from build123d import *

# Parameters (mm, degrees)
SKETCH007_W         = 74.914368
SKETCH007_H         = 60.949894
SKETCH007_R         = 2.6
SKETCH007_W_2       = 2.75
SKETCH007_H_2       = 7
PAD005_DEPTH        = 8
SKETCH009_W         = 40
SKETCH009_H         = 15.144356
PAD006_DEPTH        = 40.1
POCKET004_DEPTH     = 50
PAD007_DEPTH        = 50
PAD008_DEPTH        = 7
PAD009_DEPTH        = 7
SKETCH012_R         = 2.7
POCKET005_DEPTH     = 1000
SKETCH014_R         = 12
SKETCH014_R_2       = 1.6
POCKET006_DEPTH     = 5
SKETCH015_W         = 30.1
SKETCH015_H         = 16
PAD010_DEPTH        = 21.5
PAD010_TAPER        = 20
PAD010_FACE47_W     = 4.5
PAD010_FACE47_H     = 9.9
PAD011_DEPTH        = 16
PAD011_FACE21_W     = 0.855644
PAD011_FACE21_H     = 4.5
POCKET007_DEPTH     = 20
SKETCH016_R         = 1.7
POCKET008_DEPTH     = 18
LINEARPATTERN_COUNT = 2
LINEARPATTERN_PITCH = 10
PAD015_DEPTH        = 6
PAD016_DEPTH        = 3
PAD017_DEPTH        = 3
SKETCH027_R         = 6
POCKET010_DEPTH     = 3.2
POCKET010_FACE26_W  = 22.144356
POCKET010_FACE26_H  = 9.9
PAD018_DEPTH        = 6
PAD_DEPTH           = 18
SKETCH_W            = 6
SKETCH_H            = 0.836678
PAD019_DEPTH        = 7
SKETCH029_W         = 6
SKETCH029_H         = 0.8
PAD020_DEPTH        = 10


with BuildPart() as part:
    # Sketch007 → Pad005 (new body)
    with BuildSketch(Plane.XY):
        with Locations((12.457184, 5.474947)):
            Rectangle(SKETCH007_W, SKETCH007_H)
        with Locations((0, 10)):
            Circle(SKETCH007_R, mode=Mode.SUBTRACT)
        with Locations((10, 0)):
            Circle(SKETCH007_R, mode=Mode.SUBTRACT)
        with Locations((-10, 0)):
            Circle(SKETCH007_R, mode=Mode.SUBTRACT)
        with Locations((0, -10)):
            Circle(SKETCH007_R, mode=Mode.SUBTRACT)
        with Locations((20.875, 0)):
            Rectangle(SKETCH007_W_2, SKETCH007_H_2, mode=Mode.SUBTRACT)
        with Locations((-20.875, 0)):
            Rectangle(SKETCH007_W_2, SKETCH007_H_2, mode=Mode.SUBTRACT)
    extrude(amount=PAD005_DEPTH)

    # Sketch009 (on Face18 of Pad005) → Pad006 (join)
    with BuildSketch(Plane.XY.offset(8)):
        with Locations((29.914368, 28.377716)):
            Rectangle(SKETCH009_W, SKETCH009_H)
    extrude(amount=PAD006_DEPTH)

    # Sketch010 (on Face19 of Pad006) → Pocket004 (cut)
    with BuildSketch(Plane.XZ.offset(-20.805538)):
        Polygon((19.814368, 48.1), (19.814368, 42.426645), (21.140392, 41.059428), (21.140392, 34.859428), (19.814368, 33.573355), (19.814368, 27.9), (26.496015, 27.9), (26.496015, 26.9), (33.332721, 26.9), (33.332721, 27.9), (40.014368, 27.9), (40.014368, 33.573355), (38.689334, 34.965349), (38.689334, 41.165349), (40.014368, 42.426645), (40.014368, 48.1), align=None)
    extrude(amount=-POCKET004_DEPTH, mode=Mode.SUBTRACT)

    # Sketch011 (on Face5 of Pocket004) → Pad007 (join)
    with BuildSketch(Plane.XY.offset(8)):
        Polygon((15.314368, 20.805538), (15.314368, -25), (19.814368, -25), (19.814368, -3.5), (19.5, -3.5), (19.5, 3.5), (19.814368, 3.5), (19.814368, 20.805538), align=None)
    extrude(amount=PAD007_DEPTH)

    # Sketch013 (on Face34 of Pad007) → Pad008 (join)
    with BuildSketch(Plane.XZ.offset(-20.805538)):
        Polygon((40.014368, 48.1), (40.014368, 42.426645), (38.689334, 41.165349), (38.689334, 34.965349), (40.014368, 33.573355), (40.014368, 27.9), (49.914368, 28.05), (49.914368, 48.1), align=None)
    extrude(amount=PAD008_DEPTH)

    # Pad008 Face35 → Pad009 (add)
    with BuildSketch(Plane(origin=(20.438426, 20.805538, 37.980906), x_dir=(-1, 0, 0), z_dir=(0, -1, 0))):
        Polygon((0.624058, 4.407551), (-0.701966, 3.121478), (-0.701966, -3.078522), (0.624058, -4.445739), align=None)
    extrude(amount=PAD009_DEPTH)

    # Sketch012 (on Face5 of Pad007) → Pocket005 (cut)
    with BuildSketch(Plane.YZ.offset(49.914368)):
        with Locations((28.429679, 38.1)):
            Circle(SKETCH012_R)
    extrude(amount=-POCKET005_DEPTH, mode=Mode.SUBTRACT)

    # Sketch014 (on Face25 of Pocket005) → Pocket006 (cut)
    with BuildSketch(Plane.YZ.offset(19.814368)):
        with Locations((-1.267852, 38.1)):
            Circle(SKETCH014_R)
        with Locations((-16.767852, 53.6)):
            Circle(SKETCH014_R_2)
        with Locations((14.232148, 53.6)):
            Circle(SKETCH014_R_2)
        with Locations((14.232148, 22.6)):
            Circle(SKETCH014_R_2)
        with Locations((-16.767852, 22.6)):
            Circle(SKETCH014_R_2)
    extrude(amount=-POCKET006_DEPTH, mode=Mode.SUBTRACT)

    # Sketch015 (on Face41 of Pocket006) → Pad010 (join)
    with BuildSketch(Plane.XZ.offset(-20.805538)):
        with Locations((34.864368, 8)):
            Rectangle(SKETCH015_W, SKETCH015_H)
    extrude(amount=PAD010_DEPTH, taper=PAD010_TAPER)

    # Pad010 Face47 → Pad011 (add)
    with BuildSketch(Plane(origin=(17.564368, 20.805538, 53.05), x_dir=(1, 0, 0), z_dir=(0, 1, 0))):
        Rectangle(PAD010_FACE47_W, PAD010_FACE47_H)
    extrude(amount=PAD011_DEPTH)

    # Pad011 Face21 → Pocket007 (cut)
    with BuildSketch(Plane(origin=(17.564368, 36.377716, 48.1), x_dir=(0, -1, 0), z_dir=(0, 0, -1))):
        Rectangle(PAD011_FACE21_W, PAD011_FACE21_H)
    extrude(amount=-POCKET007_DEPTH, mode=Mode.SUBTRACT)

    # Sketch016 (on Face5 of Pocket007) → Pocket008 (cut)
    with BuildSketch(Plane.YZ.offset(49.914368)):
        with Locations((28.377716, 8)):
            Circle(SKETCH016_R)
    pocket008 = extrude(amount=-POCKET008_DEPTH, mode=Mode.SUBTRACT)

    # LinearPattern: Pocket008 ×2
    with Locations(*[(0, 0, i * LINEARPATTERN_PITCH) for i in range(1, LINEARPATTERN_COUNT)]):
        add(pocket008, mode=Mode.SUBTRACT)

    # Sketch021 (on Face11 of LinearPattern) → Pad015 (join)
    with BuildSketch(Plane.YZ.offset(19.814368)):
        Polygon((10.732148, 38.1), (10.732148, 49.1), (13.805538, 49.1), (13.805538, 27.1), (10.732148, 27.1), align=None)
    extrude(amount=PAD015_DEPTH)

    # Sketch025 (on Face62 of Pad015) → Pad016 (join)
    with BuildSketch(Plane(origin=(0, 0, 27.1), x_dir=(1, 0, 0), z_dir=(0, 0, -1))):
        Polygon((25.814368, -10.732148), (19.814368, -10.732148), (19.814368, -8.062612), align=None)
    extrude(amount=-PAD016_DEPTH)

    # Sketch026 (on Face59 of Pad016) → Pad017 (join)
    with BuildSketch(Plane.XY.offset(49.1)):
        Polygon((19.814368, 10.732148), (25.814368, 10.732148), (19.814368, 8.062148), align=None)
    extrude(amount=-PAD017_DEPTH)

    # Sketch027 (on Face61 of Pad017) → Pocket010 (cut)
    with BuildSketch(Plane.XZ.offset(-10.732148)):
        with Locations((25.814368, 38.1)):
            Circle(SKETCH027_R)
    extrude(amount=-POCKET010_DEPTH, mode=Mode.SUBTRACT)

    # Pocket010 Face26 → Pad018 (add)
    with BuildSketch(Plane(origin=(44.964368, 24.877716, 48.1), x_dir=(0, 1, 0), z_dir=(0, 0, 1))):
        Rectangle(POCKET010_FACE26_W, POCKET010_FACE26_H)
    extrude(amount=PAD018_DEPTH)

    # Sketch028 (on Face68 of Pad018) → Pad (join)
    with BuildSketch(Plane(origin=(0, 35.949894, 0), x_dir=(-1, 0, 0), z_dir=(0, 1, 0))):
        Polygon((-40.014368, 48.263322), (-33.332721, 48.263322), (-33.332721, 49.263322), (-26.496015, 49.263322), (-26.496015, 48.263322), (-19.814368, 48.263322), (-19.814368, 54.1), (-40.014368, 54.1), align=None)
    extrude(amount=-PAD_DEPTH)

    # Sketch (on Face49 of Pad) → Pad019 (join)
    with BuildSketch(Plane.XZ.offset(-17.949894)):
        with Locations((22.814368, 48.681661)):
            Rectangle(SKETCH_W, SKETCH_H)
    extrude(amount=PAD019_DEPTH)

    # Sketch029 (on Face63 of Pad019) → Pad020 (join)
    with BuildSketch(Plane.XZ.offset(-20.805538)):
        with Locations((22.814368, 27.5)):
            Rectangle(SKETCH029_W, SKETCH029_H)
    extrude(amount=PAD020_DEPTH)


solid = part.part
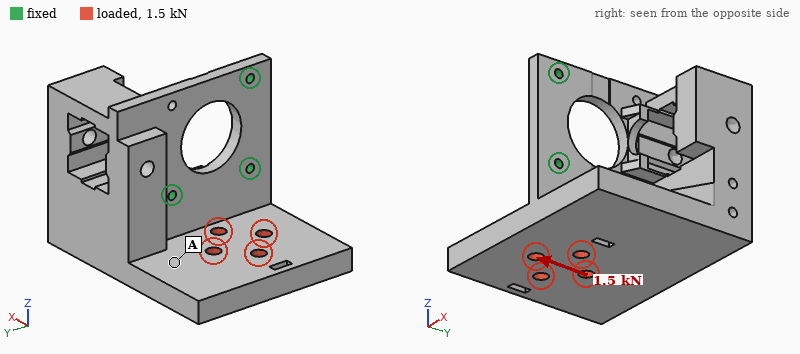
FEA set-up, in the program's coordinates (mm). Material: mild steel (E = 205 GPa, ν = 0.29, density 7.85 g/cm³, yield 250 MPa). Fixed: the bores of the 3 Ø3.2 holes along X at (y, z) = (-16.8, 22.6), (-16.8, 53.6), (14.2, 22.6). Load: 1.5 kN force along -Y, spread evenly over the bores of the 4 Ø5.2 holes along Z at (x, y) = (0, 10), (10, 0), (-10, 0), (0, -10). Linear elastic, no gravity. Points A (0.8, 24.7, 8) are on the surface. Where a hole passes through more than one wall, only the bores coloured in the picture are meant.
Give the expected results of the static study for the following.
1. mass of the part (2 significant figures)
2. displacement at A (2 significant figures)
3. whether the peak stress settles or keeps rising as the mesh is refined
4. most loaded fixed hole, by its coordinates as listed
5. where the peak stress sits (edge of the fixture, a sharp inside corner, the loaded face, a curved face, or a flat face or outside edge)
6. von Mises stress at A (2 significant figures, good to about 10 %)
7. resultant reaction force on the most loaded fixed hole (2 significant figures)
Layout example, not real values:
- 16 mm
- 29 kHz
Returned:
- 540 g
- 15 µm
- keeps rising
- (14.2, 22.6)
- edge of the fixture
- 7.9 MPa
- 1.4 kN
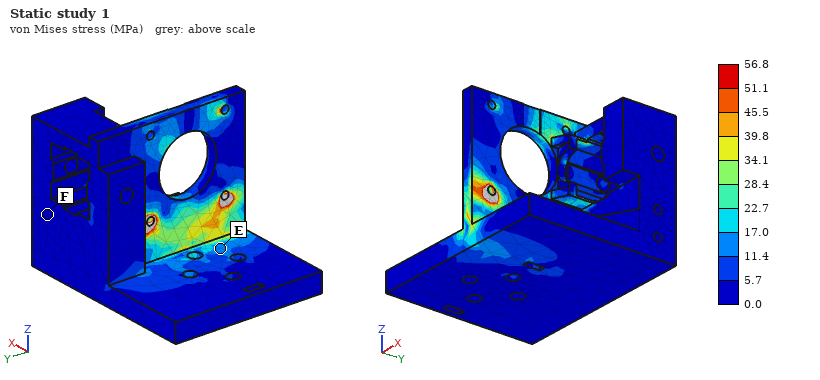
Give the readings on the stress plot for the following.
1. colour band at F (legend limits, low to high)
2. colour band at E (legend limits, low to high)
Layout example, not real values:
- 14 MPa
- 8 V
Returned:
- 0.0 to 5.7 MPa
- 11.4 to 17.0 MPa
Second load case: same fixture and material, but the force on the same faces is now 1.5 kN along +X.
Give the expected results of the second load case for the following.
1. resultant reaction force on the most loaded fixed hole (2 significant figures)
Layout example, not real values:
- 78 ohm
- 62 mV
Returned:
- 880 N
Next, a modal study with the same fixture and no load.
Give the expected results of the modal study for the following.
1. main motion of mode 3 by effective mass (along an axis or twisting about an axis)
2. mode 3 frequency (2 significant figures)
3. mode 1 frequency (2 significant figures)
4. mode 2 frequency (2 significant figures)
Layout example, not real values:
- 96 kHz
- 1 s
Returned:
- along Z
- 3700 Hz
- 1100 Hz
- 2000 Hz
